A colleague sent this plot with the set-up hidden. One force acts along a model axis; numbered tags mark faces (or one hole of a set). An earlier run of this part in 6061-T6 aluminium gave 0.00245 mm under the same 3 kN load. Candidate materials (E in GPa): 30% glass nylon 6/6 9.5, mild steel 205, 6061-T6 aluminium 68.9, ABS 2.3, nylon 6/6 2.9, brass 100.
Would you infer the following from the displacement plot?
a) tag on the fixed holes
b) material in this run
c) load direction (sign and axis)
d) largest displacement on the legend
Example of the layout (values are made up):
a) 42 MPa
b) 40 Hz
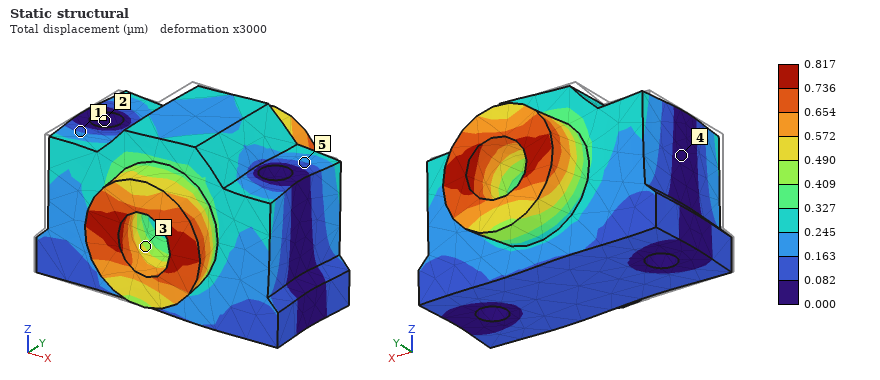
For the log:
a) 2
b) mild steel
c) +X
d) 0.817 µm
